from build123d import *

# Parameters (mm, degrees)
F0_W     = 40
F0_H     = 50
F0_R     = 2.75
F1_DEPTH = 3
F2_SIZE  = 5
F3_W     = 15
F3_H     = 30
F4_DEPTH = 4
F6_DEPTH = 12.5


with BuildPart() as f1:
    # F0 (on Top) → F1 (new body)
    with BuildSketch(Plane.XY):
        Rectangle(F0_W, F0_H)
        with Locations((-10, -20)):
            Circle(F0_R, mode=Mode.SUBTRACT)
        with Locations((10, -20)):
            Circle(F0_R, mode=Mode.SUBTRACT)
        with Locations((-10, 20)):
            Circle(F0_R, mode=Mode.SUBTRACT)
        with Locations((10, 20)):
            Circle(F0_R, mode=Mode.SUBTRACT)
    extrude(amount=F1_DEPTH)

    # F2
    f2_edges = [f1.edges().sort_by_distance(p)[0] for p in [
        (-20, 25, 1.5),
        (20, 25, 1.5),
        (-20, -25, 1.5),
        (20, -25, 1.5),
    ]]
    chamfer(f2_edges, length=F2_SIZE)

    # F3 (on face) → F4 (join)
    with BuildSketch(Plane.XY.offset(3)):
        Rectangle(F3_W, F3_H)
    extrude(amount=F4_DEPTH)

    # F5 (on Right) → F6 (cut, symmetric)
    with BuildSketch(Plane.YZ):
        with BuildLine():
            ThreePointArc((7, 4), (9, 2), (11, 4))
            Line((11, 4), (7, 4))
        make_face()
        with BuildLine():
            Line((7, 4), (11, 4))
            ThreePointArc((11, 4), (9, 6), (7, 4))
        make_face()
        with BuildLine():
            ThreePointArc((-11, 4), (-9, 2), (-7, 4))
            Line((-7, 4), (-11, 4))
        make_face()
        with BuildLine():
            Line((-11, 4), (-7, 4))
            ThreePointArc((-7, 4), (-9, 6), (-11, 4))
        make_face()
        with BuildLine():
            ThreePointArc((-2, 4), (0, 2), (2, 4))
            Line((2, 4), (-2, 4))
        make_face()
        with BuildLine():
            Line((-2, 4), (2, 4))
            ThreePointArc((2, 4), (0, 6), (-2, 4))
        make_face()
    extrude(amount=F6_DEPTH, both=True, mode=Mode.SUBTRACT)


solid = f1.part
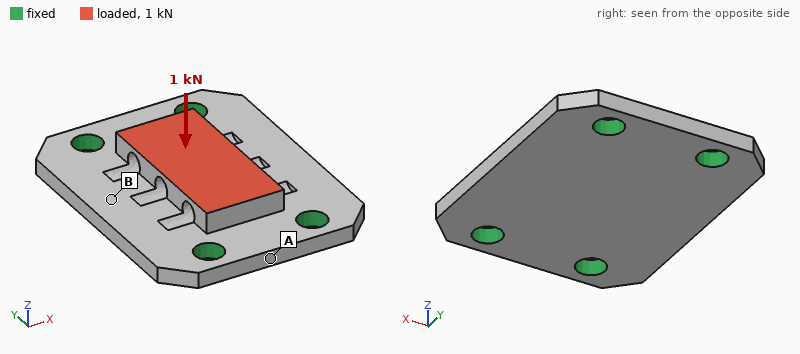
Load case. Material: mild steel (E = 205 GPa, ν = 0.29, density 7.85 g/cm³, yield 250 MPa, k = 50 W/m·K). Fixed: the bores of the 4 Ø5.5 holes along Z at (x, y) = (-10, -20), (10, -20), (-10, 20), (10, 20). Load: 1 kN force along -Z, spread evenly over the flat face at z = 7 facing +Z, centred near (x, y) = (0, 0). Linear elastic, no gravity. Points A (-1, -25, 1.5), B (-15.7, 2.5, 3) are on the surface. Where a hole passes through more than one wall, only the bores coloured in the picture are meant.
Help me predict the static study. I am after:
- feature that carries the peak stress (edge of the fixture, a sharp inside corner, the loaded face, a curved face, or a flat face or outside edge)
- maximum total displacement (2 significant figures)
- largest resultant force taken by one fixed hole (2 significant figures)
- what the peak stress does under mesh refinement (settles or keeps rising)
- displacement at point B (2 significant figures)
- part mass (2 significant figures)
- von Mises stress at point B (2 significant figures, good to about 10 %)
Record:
edge of the fixture
5.5 µm
280 N
keeps rising
3.8 µm
53 g
12 MPa
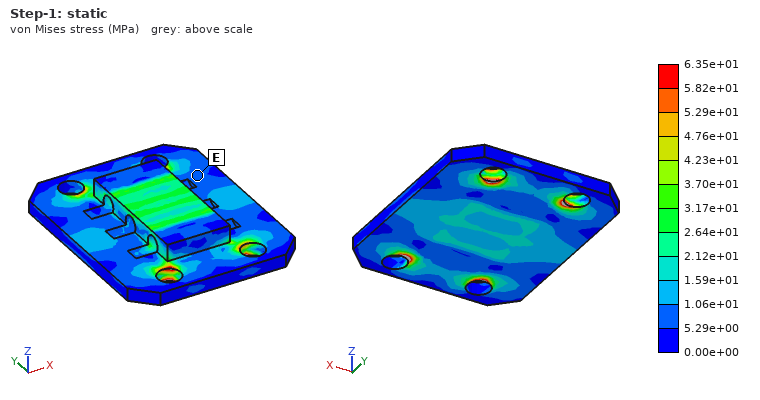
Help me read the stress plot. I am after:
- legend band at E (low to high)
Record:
5.29e+00 to 1.06e+01 MPa
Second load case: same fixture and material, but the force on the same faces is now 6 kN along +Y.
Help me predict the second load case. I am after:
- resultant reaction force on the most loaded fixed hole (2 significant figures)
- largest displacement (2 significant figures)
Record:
1.7 kN
6.9 µm
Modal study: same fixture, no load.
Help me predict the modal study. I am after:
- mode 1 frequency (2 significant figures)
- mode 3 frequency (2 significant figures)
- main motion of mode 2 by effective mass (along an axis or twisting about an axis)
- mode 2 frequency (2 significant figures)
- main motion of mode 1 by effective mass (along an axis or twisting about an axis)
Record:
12 kHz
19 kHz
twisting about Y
13 kHz
along Z
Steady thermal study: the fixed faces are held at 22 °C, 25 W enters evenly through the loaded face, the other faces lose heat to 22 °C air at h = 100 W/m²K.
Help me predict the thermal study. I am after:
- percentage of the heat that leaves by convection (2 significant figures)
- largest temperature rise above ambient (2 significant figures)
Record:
22 %
33 K
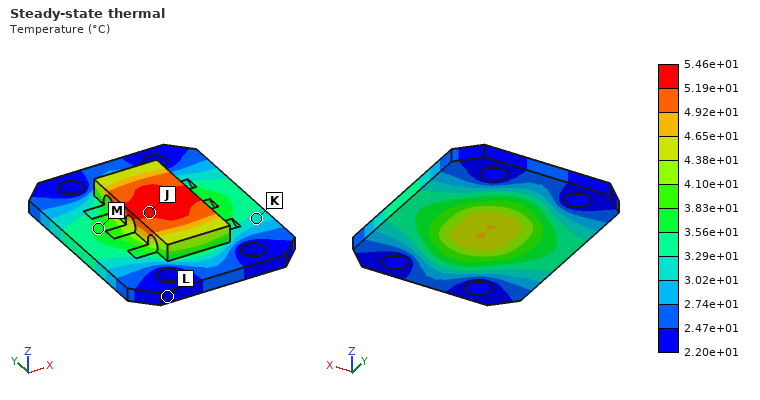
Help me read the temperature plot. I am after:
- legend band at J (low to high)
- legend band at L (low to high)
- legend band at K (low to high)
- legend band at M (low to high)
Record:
5.19e+01 to 5.46e+01 °C
2.20e+01 to 2.47e+01 °C
3.02e+01 to 3.29e+01 °C
3.56e+01 to 3.83e+01 °C
